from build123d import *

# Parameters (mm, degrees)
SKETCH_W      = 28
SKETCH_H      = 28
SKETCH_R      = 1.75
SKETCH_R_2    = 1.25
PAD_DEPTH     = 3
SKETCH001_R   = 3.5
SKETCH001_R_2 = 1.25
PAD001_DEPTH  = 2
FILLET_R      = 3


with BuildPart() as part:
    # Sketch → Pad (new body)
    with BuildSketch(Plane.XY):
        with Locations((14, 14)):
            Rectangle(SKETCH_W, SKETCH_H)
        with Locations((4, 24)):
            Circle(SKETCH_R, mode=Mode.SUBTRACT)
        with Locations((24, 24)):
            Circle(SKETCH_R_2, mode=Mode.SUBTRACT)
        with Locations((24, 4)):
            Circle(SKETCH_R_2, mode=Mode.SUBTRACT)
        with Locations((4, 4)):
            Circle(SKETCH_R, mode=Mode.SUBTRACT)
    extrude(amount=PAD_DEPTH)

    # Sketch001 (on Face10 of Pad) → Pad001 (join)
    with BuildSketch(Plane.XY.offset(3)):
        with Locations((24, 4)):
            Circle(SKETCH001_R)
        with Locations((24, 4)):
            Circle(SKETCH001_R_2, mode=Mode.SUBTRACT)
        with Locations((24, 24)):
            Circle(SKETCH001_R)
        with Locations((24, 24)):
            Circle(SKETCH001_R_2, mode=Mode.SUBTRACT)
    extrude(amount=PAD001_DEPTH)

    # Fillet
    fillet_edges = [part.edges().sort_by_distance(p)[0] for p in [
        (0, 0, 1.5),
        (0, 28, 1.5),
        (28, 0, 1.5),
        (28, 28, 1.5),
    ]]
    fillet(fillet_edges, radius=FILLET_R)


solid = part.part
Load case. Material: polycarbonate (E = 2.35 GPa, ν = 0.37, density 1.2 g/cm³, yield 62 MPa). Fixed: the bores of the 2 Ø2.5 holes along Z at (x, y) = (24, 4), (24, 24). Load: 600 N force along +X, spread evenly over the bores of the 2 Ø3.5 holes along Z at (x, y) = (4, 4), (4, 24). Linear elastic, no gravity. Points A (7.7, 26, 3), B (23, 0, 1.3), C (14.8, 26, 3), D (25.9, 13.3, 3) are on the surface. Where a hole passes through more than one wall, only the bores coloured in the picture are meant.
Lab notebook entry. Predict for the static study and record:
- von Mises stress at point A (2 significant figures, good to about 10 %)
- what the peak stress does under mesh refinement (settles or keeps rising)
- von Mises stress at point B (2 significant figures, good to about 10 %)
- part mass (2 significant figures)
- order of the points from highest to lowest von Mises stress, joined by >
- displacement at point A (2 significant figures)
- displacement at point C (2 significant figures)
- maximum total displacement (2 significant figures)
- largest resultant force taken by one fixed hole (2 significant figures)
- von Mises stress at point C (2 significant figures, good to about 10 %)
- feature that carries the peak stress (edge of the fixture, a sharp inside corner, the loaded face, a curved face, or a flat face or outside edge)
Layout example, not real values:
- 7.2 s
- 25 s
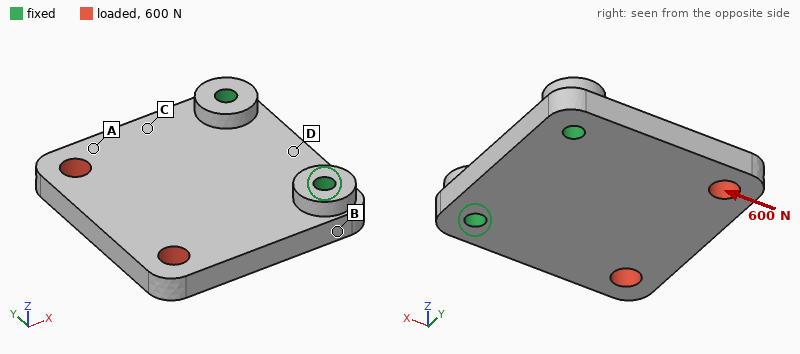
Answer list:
- 13 MPa
- keeps rising
- 6.1 MPa
- 2.9 g
- A > C > B > D
- 0.081 mm
- 0.042 mm
- 0.13 mm
- 300 N
- 10 MPa
- edge of the fixture
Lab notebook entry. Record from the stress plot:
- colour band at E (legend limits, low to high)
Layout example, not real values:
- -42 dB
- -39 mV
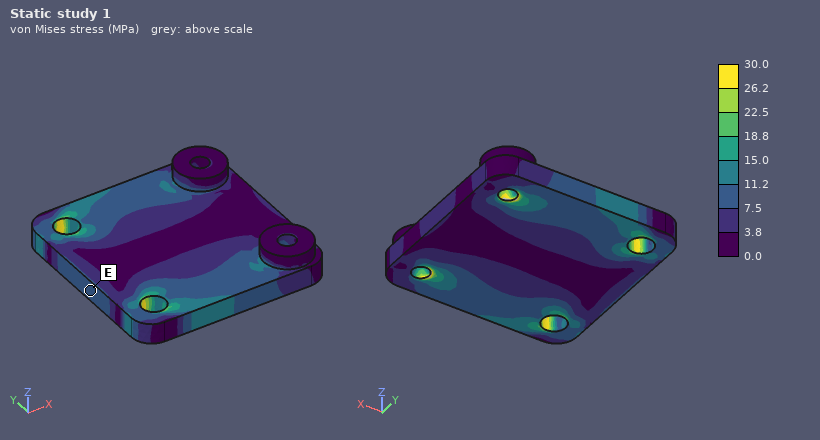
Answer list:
- 7.5 to 11.2 MPa
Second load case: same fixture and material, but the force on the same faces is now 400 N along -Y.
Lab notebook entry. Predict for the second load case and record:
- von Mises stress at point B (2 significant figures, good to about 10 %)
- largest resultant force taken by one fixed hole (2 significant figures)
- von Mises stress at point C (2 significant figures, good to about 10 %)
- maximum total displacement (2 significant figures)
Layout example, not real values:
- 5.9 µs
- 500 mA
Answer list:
- 15 MPa
- 420 N
- 11 MPa
- 0.28 mm
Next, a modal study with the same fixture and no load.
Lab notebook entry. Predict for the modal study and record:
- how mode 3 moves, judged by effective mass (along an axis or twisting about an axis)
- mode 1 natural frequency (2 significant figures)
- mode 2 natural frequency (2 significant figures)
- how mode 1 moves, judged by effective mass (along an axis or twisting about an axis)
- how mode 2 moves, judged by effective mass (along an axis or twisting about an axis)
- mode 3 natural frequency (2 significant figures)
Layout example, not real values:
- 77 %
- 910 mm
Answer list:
- along Y
- 1300 Hz
- 2800 Hz
- along Z
- twisting about X
- 6500 Hz
